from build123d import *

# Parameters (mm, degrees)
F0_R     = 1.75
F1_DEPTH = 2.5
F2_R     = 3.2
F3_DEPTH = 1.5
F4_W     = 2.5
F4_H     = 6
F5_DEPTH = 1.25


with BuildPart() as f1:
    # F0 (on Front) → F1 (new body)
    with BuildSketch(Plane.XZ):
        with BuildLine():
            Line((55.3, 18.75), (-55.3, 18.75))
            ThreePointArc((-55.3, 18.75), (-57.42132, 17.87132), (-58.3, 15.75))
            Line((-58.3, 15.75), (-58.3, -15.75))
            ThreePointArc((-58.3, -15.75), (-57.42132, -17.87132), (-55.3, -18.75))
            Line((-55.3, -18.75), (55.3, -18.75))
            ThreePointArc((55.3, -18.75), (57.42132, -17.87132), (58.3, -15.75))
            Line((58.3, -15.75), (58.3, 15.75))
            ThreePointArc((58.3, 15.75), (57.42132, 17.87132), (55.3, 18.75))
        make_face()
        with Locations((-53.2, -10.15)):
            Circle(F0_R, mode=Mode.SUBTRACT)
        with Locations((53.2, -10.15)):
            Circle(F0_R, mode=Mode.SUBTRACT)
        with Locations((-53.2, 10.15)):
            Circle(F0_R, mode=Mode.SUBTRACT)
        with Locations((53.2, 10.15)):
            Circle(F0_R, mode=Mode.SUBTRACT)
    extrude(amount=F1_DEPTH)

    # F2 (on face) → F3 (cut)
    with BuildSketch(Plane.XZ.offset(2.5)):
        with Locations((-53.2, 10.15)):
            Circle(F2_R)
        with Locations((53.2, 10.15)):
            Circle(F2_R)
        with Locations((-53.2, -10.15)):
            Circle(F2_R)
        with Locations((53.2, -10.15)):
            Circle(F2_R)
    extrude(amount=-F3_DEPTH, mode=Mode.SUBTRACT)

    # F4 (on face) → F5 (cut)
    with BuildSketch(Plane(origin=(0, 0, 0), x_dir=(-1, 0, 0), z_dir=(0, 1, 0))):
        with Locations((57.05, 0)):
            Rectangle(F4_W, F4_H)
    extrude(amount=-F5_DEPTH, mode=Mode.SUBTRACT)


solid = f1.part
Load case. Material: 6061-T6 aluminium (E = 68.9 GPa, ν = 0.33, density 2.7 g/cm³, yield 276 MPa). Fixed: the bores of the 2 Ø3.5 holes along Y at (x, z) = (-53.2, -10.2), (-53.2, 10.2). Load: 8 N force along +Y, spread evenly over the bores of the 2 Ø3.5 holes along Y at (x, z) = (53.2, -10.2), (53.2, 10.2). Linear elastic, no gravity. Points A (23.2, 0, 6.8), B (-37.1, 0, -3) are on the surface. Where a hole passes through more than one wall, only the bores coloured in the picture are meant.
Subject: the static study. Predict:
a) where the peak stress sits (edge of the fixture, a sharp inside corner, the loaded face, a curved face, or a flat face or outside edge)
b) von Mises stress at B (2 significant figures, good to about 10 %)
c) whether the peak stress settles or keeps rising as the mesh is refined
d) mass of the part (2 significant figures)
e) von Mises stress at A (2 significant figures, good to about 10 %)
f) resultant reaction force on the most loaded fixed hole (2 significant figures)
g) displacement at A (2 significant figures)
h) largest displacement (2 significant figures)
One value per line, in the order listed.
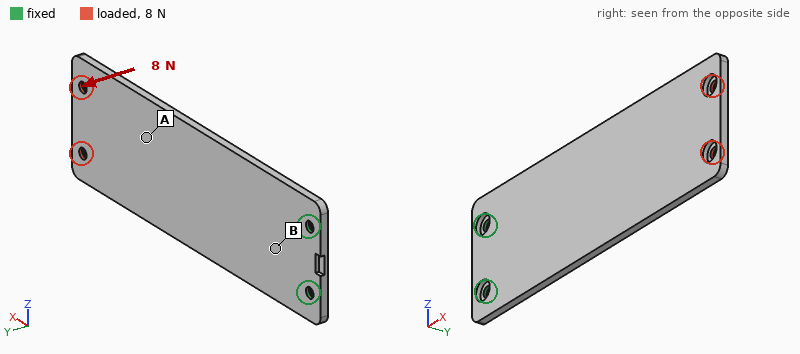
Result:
edge of the fixture
18 MPa
keeps rising
29 g
6.2 MPa
16 N
0.70 mm
1.2 mm
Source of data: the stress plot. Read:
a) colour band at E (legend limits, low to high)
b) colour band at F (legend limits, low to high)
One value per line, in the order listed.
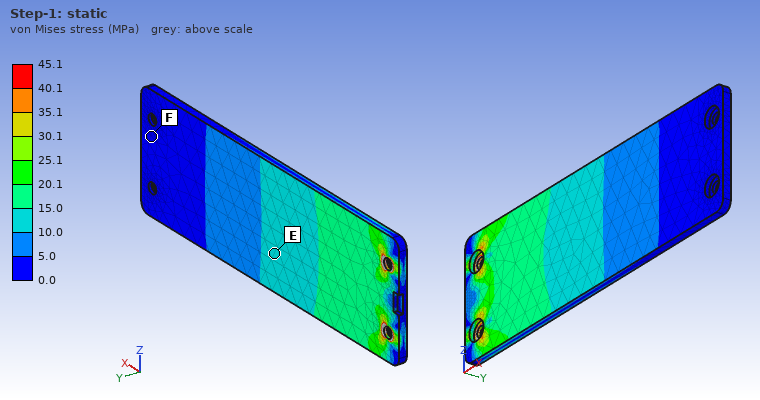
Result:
10.0 to 15.0 MPa
0.0 to 5.0 MPa
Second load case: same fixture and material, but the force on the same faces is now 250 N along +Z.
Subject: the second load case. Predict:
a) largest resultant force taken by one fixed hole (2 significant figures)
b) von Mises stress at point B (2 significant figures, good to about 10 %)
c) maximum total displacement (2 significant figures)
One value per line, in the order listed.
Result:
1.2 kN
22 MPa
0.27 mm
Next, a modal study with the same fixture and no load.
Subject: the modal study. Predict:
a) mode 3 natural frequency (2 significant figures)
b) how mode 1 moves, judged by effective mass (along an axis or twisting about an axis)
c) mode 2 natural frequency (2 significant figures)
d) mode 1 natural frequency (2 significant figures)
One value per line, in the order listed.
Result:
960 Hz
along Y
950 Hz
150 Hz
